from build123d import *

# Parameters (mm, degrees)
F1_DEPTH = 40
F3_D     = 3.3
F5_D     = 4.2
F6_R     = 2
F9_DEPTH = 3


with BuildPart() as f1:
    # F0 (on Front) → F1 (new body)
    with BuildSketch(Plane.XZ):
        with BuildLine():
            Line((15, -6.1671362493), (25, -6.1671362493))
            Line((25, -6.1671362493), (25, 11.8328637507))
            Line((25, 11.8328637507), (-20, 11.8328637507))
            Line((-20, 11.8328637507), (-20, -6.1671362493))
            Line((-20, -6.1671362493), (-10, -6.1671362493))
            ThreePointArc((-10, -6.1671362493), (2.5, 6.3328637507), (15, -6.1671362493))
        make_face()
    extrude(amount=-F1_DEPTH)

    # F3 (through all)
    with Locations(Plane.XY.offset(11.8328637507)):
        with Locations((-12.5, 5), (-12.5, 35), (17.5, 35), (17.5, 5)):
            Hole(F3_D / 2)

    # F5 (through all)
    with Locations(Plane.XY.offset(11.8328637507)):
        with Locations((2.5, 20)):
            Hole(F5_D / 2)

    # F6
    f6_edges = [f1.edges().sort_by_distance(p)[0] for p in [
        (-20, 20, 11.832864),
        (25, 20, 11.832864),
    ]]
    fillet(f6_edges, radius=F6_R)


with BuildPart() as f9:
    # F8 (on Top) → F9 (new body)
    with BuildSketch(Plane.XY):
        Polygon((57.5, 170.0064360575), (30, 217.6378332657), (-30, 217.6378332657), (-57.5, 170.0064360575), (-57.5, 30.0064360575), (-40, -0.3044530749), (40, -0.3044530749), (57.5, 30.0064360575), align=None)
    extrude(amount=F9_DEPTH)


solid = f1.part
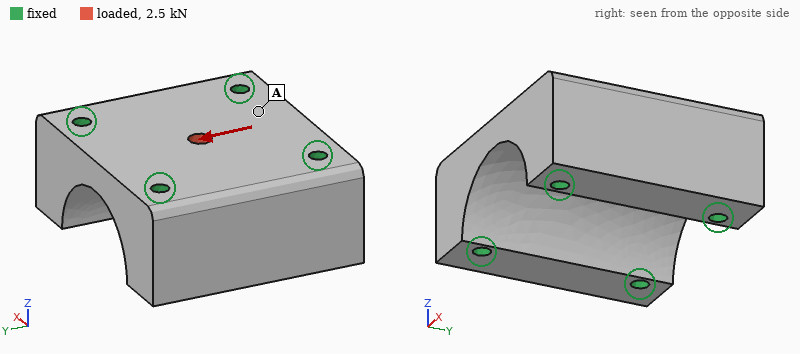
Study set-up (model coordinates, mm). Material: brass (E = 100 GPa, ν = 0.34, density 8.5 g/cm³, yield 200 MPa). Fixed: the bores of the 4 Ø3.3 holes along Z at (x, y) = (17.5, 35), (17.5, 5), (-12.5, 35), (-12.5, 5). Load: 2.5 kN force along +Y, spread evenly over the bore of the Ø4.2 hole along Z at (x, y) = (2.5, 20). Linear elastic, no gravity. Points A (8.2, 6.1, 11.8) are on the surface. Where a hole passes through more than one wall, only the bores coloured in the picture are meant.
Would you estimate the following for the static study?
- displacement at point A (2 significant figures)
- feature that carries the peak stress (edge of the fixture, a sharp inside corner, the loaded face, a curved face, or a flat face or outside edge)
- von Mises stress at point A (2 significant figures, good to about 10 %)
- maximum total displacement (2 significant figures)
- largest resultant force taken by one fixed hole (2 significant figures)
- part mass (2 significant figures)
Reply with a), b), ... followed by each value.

a) 1.1 µm
b) the loaded face
c) 6.6 MPa
d) 3.1 µm
e) 750 N
f) 190 g
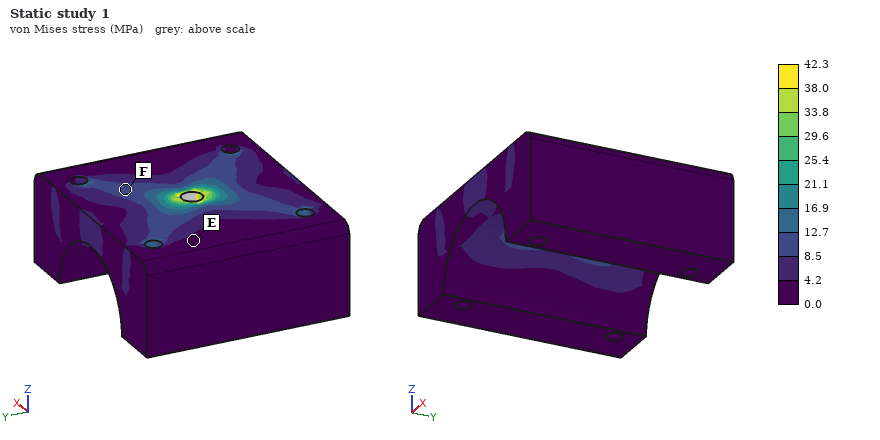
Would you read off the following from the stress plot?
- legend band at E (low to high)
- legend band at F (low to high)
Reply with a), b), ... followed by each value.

a) 0.0 to 4.2 MPa
b) 8.5 to 12.7 MPa
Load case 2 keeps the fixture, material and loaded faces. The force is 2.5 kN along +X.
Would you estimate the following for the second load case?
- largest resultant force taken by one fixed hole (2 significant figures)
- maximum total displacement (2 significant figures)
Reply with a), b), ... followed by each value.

a) 670 N
b) 3.0 µm
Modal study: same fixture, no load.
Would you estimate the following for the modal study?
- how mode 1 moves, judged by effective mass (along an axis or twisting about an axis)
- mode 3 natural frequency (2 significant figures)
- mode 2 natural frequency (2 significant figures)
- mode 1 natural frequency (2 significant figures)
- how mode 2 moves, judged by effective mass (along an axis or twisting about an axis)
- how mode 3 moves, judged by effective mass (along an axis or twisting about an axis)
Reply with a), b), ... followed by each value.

a) along Z
b) 27 kHz
c) 26 kHz
d) 23 kHz
e) along X
f) along Z
